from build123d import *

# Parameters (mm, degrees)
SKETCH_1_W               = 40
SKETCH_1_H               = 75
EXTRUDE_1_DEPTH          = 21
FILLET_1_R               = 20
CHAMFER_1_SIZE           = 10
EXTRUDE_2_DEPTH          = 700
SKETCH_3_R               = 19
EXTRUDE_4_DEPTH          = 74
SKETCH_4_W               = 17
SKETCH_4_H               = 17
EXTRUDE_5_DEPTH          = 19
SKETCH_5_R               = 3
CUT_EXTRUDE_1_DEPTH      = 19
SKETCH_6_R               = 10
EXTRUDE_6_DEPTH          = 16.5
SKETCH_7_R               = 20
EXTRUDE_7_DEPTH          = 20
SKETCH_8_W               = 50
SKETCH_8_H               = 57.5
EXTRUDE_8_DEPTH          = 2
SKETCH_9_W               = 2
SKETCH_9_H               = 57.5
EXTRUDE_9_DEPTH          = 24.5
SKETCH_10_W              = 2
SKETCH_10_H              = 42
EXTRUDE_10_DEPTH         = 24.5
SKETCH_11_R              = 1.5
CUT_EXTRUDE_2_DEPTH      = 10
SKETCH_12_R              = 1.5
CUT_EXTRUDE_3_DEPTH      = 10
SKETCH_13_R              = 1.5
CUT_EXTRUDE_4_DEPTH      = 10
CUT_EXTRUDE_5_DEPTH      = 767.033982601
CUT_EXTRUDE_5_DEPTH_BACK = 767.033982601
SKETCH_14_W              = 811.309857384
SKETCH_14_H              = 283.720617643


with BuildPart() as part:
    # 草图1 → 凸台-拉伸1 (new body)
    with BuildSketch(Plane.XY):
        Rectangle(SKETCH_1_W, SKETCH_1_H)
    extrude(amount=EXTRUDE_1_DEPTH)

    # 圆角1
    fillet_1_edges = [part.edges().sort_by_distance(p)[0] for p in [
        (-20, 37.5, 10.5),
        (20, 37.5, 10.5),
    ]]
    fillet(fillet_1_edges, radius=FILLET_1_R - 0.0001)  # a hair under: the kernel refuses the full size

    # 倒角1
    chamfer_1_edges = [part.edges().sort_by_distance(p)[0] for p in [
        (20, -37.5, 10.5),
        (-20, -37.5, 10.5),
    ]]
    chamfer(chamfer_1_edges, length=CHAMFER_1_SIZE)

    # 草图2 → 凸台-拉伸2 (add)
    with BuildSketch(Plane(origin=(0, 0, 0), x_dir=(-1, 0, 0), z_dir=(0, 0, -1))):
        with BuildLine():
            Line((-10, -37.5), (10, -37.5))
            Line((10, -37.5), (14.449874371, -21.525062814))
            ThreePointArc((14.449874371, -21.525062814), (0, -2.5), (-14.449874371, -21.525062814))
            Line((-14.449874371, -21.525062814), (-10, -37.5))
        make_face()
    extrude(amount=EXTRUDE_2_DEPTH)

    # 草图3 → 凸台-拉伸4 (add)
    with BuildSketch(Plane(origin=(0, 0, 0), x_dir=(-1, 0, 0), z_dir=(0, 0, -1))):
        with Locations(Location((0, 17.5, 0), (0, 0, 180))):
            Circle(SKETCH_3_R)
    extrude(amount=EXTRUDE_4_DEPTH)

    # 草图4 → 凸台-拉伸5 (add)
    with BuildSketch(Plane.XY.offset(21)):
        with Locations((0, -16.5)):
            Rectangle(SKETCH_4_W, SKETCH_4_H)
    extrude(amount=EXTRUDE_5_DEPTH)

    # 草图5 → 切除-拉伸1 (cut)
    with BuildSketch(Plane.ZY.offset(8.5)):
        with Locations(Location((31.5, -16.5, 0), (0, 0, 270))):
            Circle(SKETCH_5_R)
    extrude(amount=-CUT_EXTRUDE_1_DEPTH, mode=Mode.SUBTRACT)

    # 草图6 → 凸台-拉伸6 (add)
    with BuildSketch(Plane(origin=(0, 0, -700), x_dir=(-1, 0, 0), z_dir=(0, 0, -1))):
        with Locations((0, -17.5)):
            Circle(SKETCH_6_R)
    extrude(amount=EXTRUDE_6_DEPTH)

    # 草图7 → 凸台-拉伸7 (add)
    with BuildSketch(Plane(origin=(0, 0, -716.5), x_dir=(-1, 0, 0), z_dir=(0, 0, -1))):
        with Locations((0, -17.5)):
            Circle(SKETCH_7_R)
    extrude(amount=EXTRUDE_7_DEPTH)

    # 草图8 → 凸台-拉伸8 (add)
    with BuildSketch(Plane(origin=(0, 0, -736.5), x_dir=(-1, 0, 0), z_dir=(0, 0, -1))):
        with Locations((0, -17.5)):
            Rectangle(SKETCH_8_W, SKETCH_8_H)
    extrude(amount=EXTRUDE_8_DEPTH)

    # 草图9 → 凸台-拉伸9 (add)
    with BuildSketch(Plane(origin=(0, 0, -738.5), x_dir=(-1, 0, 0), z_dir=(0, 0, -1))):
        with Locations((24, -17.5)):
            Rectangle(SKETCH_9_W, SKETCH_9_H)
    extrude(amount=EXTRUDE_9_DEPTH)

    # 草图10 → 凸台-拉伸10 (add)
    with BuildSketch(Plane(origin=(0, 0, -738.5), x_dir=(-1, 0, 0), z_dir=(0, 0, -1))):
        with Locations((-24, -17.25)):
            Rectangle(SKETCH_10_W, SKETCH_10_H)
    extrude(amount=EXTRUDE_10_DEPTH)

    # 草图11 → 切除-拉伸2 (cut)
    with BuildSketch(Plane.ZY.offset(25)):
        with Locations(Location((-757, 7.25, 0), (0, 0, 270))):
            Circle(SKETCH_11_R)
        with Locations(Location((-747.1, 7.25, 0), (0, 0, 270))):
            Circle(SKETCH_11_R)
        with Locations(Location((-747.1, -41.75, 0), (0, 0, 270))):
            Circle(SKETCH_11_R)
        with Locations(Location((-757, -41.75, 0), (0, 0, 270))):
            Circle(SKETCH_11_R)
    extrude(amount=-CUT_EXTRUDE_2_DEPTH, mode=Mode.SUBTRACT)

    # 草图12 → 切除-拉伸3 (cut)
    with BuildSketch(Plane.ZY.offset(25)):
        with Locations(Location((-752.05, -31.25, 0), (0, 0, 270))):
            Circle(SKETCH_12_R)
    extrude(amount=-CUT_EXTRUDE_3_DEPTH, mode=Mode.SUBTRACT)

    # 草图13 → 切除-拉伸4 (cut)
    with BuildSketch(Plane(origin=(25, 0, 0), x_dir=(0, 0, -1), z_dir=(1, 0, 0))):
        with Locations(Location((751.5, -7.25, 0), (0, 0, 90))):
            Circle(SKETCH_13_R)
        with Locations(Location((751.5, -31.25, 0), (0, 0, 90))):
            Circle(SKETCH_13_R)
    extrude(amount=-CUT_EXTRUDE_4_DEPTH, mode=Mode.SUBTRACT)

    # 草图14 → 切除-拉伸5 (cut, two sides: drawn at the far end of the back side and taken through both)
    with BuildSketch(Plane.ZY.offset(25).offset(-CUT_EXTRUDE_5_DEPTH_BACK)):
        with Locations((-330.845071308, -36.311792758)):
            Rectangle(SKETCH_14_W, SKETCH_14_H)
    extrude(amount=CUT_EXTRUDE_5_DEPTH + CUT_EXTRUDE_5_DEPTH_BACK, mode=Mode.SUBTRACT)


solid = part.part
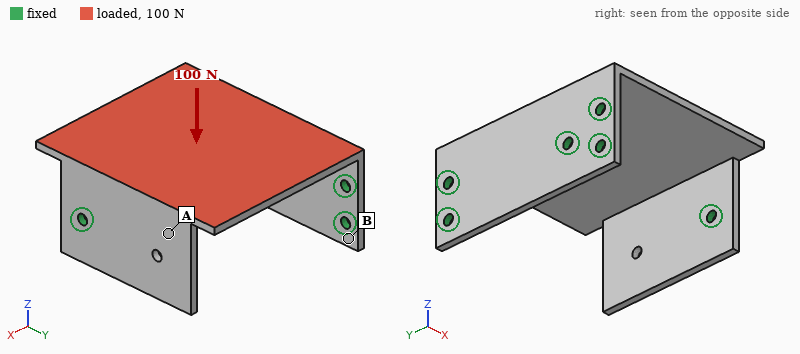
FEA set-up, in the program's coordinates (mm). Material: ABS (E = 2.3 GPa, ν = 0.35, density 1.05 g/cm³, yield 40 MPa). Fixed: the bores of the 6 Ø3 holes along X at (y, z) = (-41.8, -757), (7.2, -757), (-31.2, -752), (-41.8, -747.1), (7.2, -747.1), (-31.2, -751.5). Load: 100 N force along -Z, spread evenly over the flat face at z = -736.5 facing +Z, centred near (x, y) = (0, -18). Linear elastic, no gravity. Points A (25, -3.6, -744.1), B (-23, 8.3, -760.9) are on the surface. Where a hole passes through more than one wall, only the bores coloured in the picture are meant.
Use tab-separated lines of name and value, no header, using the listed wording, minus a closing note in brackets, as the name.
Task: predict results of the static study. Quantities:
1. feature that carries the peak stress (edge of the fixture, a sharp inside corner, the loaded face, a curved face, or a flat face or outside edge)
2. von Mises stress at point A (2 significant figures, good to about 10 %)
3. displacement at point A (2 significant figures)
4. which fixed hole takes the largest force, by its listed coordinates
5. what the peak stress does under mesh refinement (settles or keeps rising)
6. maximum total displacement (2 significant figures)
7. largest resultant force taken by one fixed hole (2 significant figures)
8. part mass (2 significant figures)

feature that carries the peak stress	edge of the fixture
von Mises stress at point A	3.3 MPa
displacement at point A	0.29 mm
which fixed hole takes the largest force, by its listed coordinates	(-31.2, -751.5)
what the peak stress does under mesh refinement	keeps rising
maximum total displacement	0.87 mm
largest resultant force taken by one fixed hole	58 N
part mass	11 g
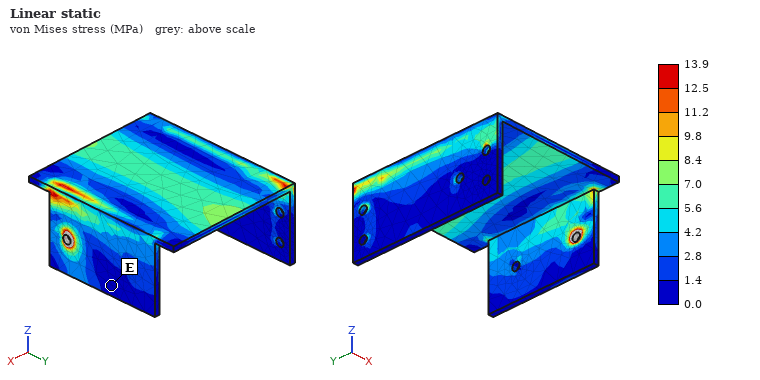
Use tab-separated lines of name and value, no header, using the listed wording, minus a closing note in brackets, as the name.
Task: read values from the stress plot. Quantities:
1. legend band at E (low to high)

legend band at E	0.0 to 1.4 MPa
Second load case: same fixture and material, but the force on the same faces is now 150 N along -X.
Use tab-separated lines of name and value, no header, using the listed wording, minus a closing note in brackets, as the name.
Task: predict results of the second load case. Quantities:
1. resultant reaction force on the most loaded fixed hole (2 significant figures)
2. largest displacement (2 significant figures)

resultant reaction force on the most loaded fixed hole	60 N
largest displacement	0.55 mm
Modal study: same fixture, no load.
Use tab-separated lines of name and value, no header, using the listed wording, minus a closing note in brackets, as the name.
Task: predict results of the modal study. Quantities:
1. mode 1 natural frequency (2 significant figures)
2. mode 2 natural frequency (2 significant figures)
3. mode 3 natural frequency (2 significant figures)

mode 1 natural frequency	770 Hz
mode 2 natural frequency	850 Hz
mode 3 natural frequency	1100 Hz
